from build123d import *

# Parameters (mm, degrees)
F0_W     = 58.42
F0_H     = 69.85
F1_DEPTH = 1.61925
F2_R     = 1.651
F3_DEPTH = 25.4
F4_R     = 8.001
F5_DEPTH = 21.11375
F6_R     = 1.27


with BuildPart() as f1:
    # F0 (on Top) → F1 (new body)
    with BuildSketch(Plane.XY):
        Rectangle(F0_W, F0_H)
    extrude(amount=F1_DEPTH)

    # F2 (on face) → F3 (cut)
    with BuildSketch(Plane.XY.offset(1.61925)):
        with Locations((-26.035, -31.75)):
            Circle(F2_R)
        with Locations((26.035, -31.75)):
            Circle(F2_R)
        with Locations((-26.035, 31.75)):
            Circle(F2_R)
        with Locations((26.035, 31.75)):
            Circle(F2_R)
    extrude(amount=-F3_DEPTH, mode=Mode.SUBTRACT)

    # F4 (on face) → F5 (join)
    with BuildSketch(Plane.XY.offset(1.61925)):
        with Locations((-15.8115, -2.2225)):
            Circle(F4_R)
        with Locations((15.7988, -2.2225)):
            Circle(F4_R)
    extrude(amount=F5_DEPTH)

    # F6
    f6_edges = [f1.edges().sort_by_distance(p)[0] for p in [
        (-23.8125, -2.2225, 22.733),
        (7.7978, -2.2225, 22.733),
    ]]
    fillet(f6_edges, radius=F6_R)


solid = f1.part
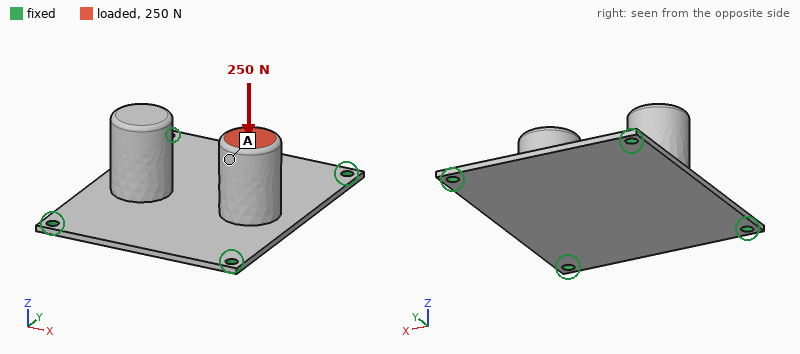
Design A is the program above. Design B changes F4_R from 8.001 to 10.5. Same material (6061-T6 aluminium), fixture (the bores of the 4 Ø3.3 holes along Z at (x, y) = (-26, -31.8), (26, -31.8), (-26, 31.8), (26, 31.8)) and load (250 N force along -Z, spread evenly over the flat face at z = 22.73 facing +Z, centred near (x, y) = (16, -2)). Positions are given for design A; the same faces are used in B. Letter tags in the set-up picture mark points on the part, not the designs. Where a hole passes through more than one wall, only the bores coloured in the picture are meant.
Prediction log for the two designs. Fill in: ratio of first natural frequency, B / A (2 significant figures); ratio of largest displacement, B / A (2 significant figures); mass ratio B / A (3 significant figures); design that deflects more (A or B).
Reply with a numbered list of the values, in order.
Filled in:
1. 0.90
2. 0.76
3. 1.41
4. A
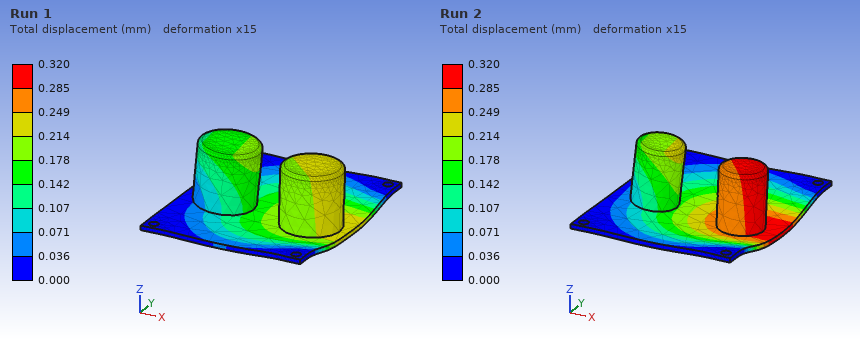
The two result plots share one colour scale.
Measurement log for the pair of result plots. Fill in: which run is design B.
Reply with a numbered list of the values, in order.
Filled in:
1. Run 1
